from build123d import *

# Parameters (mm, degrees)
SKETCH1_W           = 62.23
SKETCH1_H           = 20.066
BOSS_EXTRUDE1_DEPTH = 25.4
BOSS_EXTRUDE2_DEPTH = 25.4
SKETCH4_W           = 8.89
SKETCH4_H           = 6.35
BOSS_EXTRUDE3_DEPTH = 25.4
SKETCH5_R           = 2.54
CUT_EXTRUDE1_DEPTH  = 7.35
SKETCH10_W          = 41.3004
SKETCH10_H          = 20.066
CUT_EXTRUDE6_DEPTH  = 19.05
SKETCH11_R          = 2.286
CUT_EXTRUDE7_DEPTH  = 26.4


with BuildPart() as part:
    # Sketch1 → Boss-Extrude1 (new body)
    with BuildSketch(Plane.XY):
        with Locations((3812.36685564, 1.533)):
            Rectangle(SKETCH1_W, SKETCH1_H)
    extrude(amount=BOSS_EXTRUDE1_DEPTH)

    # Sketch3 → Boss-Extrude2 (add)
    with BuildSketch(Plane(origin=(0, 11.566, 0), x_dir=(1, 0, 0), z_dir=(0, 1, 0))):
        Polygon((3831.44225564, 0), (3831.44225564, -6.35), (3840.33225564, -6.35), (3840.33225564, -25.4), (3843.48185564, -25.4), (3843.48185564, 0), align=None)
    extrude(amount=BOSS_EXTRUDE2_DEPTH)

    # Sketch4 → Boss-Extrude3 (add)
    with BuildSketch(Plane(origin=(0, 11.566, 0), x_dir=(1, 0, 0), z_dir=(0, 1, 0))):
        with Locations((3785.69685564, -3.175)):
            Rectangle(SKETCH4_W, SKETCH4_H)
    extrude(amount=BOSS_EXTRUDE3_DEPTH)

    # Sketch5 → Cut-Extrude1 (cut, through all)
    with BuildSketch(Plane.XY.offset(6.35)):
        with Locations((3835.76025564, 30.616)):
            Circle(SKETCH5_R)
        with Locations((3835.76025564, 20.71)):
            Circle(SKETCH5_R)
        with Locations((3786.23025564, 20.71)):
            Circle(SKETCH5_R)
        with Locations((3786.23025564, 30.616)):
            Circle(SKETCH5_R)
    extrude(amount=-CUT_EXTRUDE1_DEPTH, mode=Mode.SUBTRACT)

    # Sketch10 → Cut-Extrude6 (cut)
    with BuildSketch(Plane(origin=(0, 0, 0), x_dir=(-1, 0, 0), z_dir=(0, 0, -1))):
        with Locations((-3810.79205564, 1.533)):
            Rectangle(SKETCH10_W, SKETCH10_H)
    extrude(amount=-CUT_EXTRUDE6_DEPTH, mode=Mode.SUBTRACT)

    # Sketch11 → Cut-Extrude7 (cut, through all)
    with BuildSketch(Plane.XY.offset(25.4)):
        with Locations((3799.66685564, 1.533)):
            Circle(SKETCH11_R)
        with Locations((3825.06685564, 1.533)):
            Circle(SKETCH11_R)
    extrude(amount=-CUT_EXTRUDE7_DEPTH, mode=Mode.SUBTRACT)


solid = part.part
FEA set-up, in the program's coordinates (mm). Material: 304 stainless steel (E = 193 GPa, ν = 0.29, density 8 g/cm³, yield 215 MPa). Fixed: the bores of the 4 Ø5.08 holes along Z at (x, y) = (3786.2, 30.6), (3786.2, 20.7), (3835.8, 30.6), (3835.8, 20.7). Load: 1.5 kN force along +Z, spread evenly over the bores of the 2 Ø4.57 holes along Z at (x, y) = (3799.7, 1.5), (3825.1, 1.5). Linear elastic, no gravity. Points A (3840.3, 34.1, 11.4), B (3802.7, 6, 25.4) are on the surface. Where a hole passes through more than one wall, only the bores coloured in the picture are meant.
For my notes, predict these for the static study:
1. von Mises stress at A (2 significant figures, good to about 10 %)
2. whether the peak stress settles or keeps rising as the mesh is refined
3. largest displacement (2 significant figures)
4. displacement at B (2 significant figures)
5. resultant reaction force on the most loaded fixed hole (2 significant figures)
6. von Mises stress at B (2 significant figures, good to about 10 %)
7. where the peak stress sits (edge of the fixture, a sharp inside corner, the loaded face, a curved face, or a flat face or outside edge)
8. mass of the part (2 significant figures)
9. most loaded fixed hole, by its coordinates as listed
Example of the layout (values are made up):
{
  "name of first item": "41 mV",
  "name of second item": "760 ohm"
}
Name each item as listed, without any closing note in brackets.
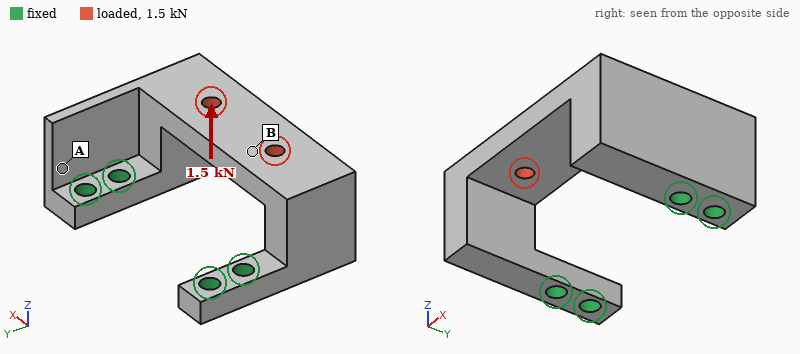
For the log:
{
  "von Mises stress at A": "18 MPa",
  "whether the peak stress settles or keeps rising as the mesh is refined": "keeps rising",
  "largest displacement": "50 µm",
  "displacement at B": "35 µm",
  "resultant reaction force on the most loaded fixed hole": "1.6 kN",
  "von Mises stress at B": "44 MPa",
  "where the peak stress sits": "edge of the fixture",
  "mass of the part": "160 g",
  "most loaded fixed hole, by its coordinates as listed": "(3835.8, 20.7)"
}
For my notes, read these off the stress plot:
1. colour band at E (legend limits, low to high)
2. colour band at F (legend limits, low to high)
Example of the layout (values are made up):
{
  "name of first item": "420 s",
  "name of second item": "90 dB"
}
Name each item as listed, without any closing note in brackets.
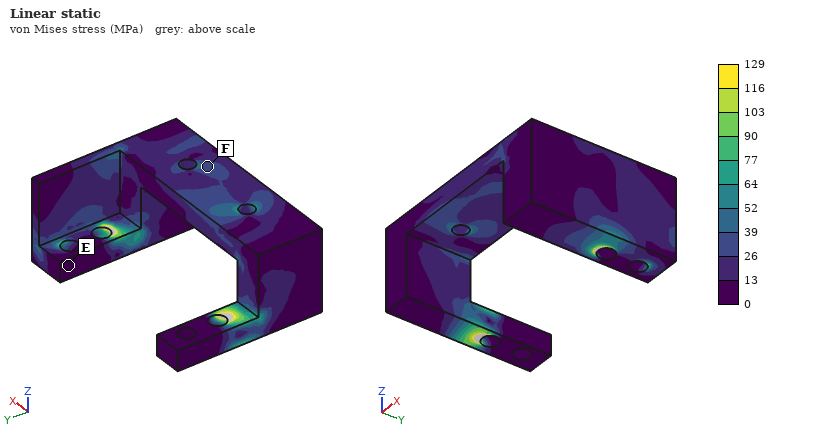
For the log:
{
  "colour band at E": "0 to 13 MPa",
  "colour band at F": "26 to 39 MPa"
}
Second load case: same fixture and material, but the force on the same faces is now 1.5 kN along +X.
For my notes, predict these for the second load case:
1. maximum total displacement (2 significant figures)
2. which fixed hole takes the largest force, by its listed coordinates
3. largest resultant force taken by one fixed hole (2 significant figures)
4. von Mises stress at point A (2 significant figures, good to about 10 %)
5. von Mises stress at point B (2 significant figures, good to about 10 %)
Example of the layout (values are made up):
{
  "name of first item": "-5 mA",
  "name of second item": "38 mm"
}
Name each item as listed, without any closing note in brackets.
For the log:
{
  "maximum total displacement": "29 µm",
  "which fixed hole takes the largest force, by its listed coordinates": "(3835.8, 20.7)",
  "largest resultant force taken by one fixed hole": "1.3 kN",
  "von Mises stress at point A": "27 MPa",
  "von Mises stress at point B": "22 MPa"
}
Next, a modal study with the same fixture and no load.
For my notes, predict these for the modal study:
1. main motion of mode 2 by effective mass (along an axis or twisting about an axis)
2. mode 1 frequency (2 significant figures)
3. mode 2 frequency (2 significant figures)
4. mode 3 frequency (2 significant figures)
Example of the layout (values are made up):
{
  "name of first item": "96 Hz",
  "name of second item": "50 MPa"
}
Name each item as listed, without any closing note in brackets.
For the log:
{
  "main motion of mode 2 by effective mass": "along X",
  "mode 1 frequency": "2700 Hz",
  "mode 2 frequency": "4300 Hz",
  "mode 3 frequency": "5400 Hz"
}
